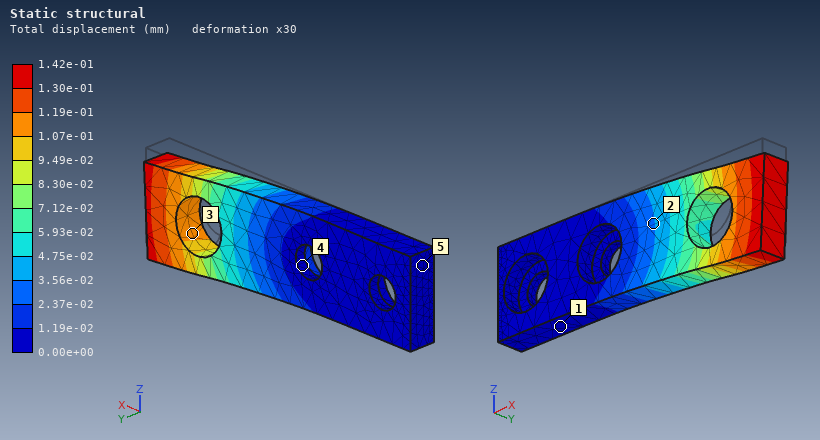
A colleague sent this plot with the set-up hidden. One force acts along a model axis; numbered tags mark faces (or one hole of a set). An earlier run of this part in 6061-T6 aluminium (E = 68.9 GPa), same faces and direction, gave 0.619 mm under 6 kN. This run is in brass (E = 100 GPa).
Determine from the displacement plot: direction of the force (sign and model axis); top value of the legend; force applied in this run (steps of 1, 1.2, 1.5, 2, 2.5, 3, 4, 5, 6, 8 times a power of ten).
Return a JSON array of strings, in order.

["-Z", "1.42e-01 mm", "2 kN"]
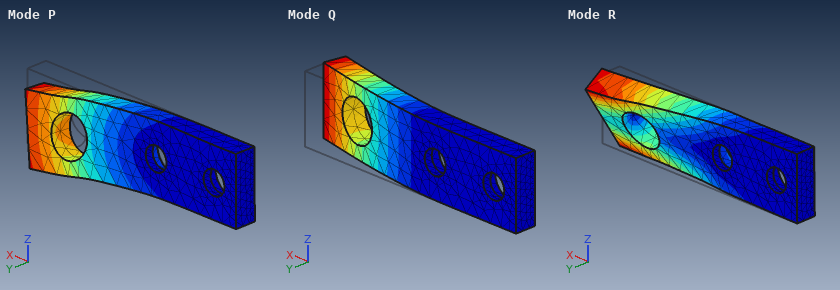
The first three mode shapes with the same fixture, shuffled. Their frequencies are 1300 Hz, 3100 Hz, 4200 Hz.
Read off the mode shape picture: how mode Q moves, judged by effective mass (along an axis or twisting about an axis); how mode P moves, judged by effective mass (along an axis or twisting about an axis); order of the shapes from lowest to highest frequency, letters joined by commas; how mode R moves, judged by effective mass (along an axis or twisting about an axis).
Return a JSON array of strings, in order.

["along Y", "along Z", "Q, P, R", "twisting about X"]
